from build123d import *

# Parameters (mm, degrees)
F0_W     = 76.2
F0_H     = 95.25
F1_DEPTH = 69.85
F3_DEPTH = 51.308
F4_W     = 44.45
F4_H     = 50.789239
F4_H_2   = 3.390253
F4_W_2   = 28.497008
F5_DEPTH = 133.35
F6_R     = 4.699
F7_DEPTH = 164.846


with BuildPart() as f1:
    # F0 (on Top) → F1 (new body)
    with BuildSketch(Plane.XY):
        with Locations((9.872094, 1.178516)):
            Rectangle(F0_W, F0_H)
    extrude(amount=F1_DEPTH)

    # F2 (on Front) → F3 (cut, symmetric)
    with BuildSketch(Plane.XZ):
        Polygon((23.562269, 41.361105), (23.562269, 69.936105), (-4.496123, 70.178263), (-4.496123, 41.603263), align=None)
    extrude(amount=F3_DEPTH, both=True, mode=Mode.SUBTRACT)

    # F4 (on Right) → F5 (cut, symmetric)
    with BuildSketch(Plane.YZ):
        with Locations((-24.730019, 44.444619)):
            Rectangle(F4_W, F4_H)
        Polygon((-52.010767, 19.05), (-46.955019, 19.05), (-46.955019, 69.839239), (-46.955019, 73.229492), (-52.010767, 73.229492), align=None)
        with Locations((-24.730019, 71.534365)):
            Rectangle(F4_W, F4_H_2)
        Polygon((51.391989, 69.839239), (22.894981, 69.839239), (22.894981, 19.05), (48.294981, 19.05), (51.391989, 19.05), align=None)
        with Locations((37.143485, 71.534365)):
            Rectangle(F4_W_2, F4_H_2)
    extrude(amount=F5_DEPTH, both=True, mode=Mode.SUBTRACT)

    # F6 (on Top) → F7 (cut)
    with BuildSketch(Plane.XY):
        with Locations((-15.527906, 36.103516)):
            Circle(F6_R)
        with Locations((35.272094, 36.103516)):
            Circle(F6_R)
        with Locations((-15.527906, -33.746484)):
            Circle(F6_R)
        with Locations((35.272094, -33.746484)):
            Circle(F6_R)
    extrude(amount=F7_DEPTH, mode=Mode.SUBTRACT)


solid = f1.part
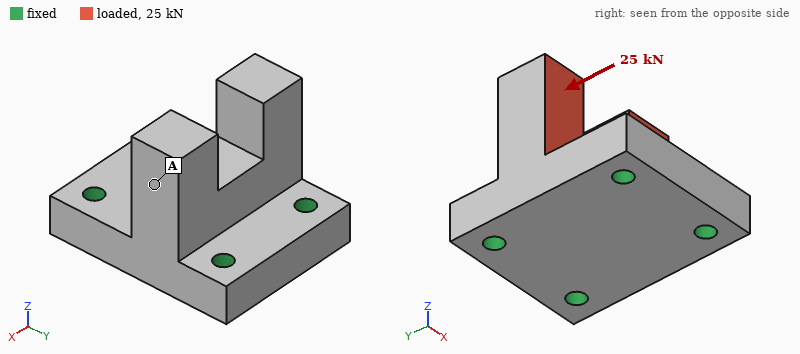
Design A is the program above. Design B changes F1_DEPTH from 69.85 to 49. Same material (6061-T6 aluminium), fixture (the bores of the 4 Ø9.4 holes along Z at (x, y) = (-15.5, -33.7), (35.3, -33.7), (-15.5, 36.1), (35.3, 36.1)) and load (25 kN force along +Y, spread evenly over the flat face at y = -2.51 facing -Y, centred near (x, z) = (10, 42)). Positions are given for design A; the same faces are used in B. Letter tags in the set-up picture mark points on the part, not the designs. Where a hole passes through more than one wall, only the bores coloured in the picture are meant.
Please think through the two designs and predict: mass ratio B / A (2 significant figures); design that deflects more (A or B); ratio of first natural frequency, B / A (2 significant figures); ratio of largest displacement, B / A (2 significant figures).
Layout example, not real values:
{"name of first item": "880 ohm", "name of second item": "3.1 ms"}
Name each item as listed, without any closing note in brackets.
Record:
{"mass ratio B / A": "0.88", "design that deflects more": "A", "ratio of first natural frequency, B / A": "1.7", "ratio of largest displacement, B / A": "0.38"}
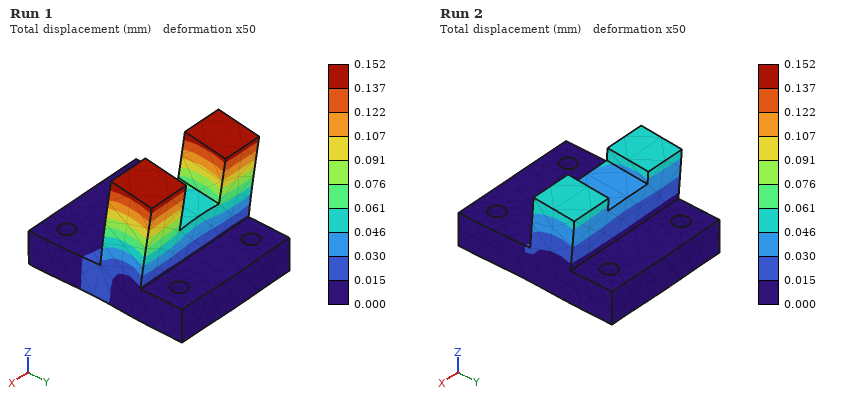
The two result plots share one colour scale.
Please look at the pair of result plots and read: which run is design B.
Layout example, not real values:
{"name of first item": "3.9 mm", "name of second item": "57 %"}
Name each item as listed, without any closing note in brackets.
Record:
{"which run is design B": "Run 2"}
